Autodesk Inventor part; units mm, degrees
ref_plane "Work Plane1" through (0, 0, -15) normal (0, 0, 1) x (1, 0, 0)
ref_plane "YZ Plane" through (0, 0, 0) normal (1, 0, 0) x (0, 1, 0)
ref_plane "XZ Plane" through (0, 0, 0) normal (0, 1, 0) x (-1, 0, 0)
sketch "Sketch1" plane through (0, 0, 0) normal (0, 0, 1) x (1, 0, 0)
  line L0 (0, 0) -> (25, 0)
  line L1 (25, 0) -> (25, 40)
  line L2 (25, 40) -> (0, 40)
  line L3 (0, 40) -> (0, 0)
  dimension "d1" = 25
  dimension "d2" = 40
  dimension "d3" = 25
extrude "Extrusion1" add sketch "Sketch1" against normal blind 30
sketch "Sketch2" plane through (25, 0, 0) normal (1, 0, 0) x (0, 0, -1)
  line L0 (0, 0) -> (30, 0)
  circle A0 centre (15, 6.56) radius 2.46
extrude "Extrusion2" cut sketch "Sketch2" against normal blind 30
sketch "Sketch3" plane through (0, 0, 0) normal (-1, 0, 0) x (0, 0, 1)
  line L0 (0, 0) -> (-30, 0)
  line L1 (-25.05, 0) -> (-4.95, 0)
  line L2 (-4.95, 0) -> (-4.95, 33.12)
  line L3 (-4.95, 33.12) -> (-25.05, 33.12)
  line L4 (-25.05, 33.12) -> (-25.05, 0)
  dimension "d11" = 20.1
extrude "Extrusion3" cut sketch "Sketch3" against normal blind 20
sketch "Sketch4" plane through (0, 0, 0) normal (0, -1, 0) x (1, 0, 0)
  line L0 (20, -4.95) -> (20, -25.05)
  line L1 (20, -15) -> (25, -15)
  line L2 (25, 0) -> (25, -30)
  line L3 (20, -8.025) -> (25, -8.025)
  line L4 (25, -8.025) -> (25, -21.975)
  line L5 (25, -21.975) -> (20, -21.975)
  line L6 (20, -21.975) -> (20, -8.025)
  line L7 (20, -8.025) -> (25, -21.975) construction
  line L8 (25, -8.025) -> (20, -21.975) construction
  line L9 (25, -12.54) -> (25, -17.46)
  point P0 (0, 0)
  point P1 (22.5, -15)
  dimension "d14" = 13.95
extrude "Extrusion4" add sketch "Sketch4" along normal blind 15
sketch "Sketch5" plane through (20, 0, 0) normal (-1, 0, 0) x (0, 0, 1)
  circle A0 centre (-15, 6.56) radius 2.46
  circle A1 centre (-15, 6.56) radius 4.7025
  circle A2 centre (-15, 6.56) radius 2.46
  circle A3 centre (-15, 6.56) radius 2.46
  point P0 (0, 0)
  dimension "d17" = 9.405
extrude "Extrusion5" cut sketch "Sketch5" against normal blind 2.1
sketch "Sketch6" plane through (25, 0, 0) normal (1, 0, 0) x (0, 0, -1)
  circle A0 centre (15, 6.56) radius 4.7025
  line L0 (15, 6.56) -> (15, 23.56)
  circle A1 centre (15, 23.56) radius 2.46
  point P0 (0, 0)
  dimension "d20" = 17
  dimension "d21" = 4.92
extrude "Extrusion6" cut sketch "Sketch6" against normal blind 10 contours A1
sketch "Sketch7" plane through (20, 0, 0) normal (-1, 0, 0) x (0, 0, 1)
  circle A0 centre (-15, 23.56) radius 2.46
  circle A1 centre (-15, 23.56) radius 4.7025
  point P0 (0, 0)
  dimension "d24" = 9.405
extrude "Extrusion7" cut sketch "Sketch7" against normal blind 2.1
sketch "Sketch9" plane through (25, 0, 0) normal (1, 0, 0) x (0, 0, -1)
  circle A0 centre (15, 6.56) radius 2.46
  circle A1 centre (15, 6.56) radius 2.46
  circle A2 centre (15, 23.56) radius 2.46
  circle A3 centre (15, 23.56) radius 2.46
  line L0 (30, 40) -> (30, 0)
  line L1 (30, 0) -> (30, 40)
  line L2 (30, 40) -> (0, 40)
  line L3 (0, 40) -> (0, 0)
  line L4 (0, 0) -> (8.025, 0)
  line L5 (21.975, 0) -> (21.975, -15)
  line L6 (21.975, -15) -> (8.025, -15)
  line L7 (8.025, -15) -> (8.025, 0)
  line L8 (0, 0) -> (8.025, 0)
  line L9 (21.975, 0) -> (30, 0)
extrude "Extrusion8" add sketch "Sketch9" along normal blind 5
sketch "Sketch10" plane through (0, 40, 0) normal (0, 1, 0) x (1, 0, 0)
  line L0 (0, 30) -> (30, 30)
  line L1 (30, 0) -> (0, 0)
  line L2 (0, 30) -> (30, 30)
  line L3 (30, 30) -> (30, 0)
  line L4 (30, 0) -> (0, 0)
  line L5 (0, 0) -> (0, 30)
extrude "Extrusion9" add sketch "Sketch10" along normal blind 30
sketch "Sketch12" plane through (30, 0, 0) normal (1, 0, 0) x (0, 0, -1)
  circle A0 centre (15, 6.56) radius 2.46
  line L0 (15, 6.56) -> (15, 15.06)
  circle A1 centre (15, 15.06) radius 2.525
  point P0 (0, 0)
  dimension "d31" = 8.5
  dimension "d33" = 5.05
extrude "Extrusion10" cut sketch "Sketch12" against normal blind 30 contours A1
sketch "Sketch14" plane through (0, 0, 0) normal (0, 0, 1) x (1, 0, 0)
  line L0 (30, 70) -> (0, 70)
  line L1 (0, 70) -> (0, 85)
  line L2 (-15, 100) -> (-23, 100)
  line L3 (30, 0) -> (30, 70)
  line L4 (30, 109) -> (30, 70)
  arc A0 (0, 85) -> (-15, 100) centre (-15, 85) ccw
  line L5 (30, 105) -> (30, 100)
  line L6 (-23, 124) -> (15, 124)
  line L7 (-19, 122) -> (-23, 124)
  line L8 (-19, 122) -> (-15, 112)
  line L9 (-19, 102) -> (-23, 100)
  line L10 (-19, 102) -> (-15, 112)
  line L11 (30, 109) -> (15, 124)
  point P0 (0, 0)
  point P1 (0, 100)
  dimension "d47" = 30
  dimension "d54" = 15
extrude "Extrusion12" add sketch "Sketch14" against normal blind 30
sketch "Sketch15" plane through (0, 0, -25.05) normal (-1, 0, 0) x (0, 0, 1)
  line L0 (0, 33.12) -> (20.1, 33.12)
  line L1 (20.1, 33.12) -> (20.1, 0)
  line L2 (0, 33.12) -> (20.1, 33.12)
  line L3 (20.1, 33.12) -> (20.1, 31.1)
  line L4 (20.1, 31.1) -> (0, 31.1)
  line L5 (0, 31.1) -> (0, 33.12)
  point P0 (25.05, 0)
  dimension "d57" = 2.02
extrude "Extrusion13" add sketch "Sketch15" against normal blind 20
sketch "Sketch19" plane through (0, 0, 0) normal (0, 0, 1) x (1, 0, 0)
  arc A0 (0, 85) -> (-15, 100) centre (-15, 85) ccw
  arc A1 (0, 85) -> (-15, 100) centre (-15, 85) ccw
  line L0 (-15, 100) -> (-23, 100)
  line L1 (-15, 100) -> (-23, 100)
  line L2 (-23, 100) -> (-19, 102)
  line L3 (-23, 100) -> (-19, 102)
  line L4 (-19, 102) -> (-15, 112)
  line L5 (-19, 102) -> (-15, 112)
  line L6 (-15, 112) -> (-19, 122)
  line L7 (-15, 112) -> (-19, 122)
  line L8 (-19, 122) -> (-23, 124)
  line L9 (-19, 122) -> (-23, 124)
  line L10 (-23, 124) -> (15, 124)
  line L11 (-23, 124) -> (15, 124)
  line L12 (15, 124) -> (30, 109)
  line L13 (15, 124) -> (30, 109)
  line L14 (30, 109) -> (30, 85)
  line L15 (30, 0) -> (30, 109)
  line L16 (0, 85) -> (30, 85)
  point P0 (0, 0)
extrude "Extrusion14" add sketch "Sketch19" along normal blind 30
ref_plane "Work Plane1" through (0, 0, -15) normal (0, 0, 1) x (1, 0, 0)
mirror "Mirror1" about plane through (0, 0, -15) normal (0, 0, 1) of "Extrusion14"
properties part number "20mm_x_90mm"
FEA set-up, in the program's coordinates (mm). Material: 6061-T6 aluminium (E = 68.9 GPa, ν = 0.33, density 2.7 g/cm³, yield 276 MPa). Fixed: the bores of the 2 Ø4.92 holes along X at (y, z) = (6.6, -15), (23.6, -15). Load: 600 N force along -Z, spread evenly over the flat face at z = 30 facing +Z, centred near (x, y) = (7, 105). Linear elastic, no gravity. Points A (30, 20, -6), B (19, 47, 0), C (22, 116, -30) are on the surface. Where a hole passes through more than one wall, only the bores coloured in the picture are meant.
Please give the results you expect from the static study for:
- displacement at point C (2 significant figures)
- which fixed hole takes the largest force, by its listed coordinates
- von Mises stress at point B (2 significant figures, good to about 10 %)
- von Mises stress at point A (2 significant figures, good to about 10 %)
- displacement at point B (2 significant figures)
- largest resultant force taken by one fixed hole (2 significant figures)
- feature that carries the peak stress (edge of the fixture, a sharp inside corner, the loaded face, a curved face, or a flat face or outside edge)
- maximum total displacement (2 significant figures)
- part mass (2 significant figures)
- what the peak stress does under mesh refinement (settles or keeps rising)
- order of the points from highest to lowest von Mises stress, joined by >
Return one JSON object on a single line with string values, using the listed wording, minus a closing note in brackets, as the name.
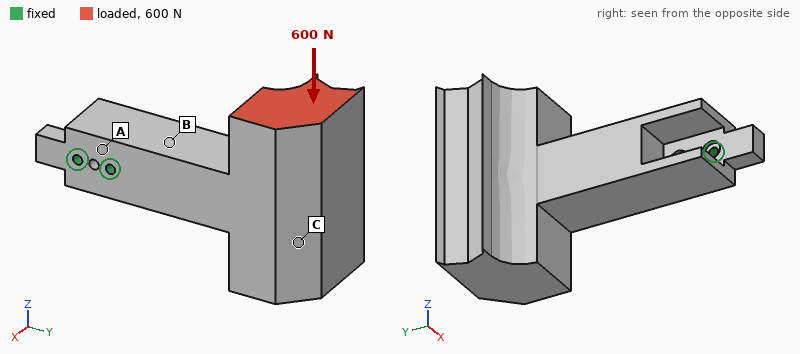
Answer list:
{"displacement at point C": "0.091 mm", "which fixed hole takes the largest force, by its listed coordinates": "(23.6, -15)", "von Mises stress at point B": "8.6 MPa", "von Mises stress at point A": "17 MPa", "displacement at point B": "0.025 mm", "largest resultant force taken by one fixed hole": "2.7 kN", "feature that carries the peak stress": "edge of the fixture", "maximum total displacement": "0.13 mm", "part mass": "550 g", "what the peak stress does under mesh refinement": "keeps rising", "order of the points from highest to lowest von Mises stress, joined by >": "A > B > C"}
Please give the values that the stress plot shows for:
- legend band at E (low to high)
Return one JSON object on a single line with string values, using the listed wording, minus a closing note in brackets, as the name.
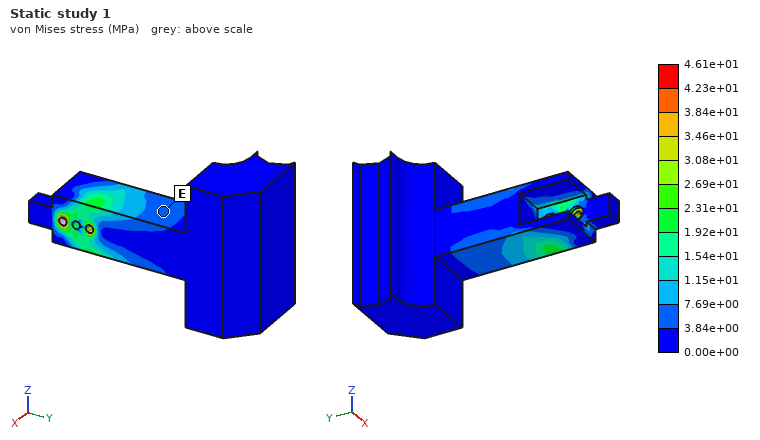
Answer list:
{"legend band at E": "3.84e+00 to 7.69e+00 MPa"}
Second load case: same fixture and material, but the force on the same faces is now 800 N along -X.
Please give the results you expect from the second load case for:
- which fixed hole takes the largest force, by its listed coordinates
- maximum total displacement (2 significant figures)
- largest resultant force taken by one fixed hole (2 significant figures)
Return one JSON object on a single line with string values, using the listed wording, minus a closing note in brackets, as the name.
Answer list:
{"which fixed hole takes the largest force, by its listed coordinates": "(23.6, -15)", "maximum total displacement": "0.32 mm", "largest resultant force taken by one fixed hole": "3.4 kN"}
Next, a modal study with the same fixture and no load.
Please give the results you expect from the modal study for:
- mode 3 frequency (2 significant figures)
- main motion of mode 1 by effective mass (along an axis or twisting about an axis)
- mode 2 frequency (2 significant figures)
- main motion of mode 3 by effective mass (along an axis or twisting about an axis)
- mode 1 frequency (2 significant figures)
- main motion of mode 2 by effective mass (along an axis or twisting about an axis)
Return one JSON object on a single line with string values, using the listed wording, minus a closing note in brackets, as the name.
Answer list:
{"mode 3 frequency": "1100 Hz", "main motion of mode 1 by effective mass": "along X", "mode 2 frequency": "630 Hz", "main motion of mode 3 by effective mass": "twisting about Y", "mode 1 frequency": "570 Hz", "main motion of mode 2 by effective mass": "along Z"}
